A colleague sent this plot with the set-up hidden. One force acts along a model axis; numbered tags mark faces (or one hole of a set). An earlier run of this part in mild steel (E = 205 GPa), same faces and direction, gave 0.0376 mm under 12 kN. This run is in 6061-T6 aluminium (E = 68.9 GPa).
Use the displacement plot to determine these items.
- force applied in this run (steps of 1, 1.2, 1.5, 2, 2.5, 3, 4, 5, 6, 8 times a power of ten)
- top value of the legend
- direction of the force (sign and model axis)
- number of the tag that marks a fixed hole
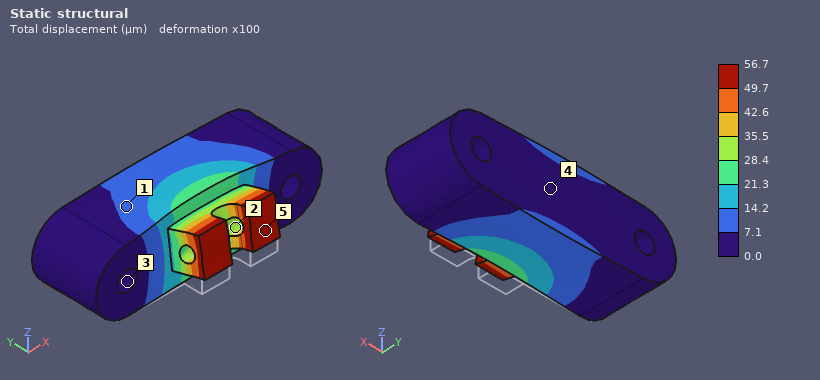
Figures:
6 kN
56.7 µm
+Z
3
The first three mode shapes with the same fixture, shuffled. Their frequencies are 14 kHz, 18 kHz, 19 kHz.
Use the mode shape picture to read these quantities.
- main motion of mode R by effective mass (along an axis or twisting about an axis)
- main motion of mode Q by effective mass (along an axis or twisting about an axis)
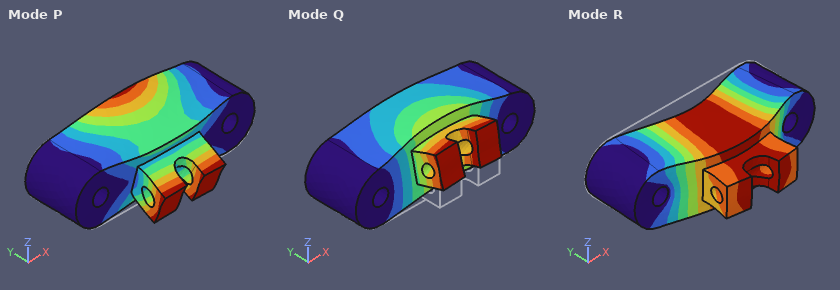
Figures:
along Y
along Z
